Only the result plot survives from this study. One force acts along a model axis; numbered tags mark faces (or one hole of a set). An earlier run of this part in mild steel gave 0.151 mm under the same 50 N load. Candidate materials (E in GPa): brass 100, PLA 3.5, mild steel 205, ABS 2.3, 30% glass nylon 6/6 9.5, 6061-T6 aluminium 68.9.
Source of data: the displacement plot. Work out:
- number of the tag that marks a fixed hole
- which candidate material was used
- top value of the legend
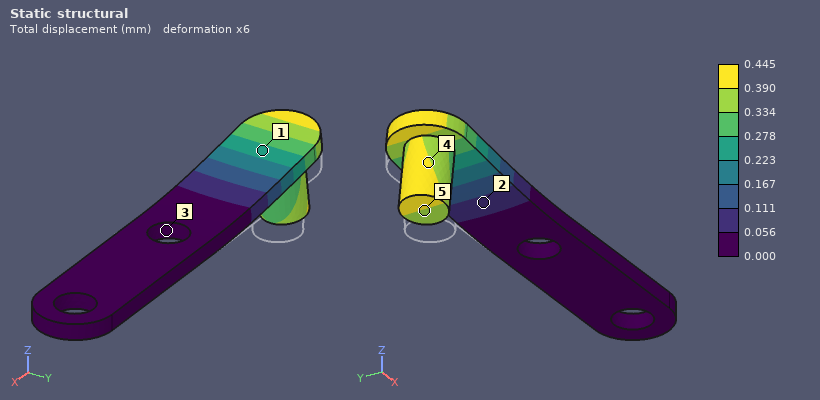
3
6061-T6 aluminium
0.445 mm
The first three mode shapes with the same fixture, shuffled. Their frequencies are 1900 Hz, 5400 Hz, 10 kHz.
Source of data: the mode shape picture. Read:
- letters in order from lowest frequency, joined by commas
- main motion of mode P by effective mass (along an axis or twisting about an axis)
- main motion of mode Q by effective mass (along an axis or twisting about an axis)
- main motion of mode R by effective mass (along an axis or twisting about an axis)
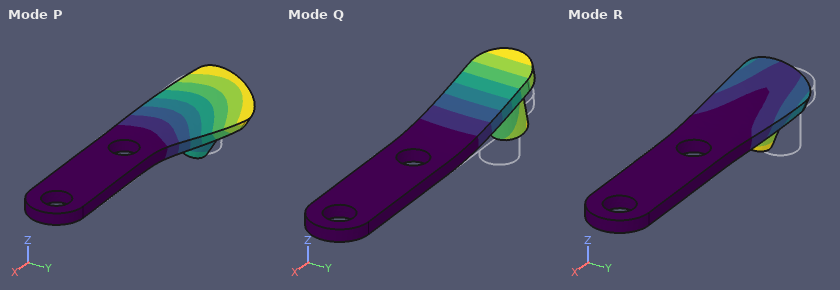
Q, R, P
along Y
along Z
along Y
